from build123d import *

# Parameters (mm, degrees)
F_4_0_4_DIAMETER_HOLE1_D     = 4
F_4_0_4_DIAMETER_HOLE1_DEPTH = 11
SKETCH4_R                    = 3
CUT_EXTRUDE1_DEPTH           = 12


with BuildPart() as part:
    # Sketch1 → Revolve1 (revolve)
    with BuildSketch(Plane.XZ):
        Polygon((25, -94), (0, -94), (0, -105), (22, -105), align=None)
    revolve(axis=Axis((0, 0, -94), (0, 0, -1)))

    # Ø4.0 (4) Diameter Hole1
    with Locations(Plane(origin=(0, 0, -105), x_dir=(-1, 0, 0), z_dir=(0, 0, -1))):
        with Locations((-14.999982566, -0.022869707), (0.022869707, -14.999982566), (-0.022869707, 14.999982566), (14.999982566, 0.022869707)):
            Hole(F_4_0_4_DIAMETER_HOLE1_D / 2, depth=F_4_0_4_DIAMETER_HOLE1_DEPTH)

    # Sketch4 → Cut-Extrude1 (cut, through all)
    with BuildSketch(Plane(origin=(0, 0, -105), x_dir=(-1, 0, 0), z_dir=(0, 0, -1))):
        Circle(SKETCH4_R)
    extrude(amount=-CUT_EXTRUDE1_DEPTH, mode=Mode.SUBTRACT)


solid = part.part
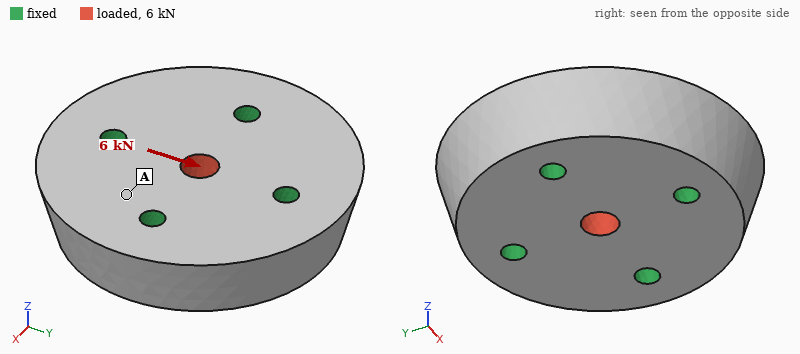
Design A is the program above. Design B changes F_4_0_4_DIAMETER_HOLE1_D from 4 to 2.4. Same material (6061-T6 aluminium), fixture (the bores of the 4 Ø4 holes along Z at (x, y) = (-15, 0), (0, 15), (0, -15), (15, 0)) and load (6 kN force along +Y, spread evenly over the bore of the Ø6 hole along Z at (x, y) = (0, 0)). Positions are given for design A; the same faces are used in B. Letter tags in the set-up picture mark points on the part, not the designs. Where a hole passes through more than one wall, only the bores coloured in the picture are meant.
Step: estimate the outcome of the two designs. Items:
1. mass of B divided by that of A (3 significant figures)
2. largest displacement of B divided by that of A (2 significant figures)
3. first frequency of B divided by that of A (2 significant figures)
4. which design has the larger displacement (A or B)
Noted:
1.02
1.1
0.87
B
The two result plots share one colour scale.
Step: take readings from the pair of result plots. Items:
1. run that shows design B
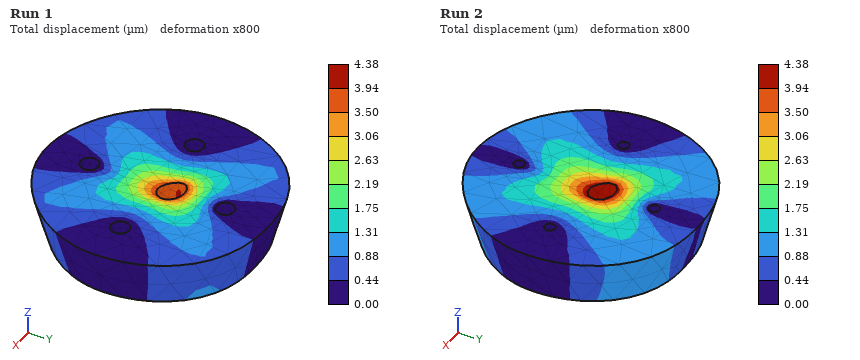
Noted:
Run 2
